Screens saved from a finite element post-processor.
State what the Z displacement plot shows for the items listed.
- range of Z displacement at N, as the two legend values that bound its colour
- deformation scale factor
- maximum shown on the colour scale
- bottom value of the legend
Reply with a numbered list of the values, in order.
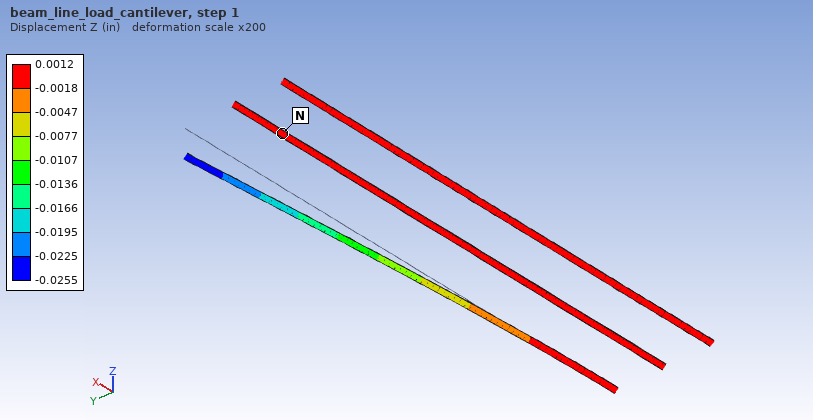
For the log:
1. -0.0018 to 0.0012 in
2. 200
3. 0.0012 in
4. -0.0255 in
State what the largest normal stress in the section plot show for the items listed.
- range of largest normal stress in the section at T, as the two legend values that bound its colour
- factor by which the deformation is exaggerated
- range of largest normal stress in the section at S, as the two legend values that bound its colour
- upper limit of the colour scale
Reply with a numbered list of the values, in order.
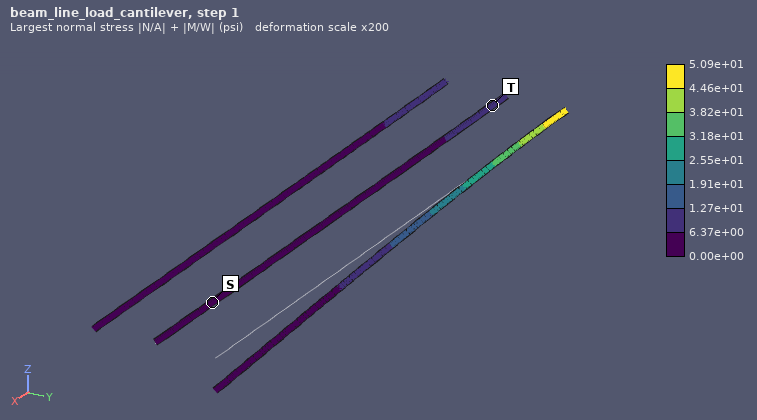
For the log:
1. 6.37e+00 to 1.27e+01 psi
2. 200
3. 0.00e+00 to 6.37e+00 psi
4. 5.09e+01 psi
